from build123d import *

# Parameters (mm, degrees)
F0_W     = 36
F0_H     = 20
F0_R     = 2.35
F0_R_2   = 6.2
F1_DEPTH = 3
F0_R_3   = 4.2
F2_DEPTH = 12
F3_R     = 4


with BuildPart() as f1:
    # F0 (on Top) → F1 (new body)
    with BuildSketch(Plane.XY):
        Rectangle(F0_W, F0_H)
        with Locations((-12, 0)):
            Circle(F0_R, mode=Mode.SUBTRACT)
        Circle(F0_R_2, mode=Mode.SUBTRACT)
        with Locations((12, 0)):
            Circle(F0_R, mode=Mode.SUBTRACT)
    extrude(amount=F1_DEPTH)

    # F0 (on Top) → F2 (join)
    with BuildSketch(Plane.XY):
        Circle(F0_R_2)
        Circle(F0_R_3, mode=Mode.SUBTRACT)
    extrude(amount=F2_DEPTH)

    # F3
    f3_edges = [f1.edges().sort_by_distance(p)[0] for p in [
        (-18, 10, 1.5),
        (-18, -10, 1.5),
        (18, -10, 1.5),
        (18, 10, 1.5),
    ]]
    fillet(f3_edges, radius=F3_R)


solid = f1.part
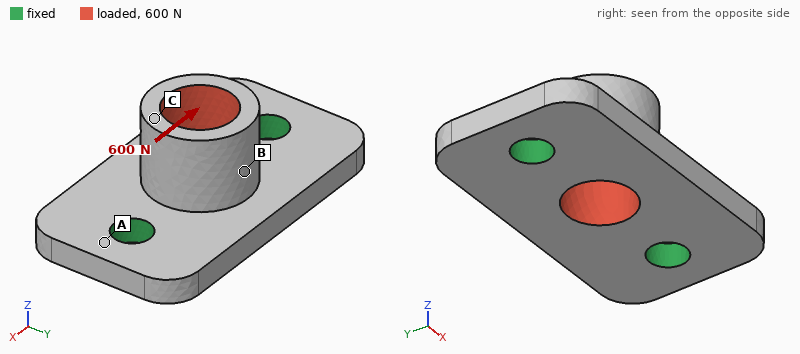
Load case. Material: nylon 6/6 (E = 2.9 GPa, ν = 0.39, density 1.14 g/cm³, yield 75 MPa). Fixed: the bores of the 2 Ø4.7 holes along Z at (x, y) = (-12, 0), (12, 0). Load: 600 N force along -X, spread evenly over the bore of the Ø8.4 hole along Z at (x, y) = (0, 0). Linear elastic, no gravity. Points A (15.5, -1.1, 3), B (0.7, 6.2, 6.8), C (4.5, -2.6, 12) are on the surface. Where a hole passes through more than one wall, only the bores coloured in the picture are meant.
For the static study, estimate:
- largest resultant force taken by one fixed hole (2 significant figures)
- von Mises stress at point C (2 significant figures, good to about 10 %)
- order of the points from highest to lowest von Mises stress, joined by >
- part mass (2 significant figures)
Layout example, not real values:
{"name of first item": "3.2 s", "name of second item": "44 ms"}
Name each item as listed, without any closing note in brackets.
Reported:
{"largest resultant force taken by one fixed hole": "340 N", "von Mises stress at point C": "6.8 MPa", "order of the points from highest to lowest von Mises stress, joined by >": "B > C > A", "part mass": "2.8 g"}
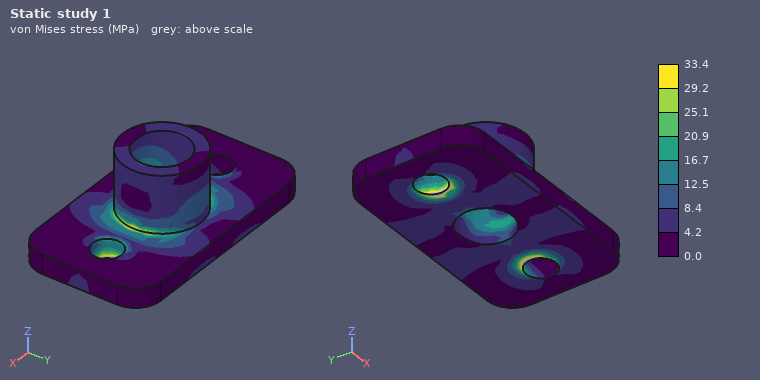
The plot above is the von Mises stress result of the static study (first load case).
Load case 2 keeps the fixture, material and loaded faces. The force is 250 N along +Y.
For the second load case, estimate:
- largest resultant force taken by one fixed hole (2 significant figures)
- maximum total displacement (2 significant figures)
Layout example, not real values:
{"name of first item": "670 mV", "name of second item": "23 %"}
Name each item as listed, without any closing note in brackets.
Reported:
{"largest resultant force taken by one fixed hole": "130 N", "maximum total displacement": "0.26 mm"}
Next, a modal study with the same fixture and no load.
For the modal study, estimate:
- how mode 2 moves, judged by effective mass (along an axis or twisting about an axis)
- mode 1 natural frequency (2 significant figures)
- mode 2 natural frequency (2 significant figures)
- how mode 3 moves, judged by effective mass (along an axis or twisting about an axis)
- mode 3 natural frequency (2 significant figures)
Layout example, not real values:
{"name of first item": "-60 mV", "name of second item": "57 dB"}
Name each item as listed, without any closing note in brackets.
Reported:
{"how mode 2 moves, judged by effective mass": "along Z", "mode 1 natural frequency": "4700 Hz", "mode 2 natural frequency": "7500 Hz", "how mode 3 moves, judged by effective mass": "along X", "mode 3 natural frequency": "10 kHz"}
